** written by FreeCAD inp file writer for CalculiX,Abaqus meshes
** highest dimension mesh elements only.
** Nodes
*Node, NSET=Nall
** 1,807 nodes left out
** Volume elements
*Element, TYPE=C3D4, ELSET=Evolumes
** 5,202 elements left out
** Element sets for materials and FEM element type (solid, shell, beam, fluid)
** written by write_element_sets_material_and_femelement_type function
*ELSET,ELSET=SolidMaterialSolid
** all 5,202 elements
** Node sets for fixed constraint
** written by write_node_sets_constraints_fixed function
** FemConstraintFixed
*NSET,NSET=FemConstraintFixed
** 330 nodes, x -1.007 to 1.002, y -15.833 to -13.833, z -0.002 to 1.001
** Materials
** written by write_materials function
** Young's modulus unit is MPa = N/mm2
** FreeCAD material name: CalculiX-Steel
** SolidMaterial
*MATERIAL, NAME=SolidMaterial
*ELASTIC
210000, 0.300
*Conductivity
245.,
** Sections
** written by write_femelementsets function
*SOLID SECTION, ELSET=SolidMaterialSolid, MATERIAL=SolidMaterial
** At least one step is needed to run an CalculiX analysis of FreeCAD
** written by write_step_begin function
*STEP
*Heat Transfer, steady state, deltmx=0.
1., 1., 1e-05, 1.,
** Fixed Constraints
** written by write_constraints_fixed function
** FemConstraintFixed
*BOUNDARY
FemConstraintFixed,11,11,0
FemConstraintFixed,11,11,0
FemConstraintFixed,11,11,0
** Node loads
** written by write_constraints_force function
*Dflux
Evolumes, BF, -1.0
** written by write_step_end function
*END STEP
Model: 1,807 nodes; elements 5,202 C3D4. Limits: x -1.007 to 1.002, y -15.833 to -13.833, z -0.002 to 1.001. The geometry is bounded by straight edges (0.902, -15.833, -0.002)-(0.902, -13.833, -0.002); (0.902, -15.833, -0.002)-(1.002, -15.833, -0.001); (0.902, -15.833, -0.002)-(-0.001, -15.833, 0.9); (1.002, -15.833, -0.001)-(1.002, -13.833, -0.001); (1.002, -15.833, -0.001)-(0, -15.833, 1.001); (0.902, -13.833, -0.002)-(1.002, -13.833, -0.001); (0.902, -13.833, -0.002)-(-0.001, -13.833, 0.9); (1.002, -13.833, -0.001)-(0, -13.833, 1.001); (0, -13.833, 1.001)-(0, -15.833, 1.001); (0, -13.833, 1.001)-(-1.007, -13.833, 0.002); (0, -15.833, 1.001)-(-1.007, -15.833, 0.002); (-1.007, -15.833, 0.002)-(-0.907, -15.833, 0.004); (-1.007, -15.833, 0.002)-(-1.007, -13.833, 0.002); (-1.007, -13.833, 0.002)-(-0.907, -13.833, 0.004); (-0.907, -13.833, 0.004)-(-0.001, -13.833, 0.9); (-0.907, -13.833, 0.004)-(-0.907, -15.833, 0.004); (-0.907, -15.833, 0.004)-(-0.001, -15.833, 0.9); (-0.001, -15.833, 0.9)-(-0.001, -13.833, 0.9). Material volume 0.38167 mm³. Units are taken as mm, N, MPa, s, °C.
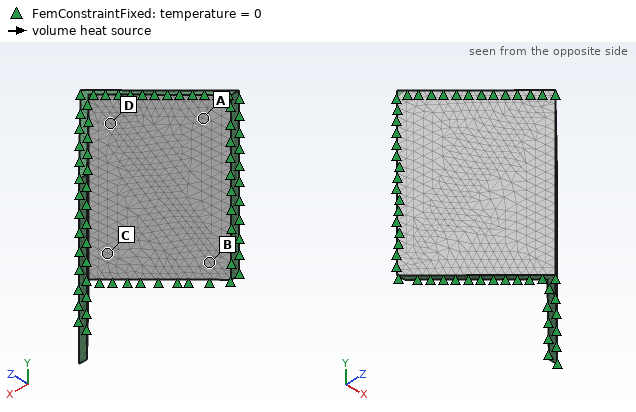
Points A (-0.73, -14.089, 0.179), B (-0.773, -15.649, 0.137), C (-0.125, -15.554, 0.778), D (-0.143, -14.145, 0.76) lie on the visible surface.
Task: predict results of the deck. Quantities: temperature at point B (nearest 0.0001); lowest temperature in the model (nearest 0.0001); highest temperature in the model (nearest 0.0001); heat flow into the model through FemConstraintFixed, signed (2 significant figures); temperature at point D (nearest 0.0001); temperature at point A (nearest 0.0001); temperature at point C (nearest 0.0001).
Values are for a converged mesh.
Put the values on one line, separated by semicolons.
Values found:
-0.0002 °C; -0.0015 °C; 0.0000 °C; 0.38 mW; -0.0008 °C; -0.0003 °C; -0.0008 °C
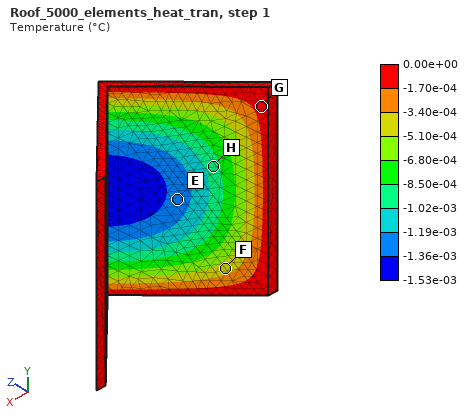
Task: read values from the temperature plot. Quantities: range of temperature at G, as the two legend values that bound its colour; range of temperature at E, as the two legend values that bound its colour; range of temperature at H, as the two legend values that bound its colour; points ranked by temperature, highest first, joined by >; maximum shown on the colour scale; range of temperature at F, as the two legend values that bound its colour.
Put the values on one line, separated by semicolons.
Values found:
-1.70e-04 to 0.00e+00 °C; -1.36e-03 to -1.19e-03 °C; -1.02e-03 to -8.50e-04 °C; G > F > H > E; 0.00e+00 °C; -5.10e-04 to -3.40e-04 °C
